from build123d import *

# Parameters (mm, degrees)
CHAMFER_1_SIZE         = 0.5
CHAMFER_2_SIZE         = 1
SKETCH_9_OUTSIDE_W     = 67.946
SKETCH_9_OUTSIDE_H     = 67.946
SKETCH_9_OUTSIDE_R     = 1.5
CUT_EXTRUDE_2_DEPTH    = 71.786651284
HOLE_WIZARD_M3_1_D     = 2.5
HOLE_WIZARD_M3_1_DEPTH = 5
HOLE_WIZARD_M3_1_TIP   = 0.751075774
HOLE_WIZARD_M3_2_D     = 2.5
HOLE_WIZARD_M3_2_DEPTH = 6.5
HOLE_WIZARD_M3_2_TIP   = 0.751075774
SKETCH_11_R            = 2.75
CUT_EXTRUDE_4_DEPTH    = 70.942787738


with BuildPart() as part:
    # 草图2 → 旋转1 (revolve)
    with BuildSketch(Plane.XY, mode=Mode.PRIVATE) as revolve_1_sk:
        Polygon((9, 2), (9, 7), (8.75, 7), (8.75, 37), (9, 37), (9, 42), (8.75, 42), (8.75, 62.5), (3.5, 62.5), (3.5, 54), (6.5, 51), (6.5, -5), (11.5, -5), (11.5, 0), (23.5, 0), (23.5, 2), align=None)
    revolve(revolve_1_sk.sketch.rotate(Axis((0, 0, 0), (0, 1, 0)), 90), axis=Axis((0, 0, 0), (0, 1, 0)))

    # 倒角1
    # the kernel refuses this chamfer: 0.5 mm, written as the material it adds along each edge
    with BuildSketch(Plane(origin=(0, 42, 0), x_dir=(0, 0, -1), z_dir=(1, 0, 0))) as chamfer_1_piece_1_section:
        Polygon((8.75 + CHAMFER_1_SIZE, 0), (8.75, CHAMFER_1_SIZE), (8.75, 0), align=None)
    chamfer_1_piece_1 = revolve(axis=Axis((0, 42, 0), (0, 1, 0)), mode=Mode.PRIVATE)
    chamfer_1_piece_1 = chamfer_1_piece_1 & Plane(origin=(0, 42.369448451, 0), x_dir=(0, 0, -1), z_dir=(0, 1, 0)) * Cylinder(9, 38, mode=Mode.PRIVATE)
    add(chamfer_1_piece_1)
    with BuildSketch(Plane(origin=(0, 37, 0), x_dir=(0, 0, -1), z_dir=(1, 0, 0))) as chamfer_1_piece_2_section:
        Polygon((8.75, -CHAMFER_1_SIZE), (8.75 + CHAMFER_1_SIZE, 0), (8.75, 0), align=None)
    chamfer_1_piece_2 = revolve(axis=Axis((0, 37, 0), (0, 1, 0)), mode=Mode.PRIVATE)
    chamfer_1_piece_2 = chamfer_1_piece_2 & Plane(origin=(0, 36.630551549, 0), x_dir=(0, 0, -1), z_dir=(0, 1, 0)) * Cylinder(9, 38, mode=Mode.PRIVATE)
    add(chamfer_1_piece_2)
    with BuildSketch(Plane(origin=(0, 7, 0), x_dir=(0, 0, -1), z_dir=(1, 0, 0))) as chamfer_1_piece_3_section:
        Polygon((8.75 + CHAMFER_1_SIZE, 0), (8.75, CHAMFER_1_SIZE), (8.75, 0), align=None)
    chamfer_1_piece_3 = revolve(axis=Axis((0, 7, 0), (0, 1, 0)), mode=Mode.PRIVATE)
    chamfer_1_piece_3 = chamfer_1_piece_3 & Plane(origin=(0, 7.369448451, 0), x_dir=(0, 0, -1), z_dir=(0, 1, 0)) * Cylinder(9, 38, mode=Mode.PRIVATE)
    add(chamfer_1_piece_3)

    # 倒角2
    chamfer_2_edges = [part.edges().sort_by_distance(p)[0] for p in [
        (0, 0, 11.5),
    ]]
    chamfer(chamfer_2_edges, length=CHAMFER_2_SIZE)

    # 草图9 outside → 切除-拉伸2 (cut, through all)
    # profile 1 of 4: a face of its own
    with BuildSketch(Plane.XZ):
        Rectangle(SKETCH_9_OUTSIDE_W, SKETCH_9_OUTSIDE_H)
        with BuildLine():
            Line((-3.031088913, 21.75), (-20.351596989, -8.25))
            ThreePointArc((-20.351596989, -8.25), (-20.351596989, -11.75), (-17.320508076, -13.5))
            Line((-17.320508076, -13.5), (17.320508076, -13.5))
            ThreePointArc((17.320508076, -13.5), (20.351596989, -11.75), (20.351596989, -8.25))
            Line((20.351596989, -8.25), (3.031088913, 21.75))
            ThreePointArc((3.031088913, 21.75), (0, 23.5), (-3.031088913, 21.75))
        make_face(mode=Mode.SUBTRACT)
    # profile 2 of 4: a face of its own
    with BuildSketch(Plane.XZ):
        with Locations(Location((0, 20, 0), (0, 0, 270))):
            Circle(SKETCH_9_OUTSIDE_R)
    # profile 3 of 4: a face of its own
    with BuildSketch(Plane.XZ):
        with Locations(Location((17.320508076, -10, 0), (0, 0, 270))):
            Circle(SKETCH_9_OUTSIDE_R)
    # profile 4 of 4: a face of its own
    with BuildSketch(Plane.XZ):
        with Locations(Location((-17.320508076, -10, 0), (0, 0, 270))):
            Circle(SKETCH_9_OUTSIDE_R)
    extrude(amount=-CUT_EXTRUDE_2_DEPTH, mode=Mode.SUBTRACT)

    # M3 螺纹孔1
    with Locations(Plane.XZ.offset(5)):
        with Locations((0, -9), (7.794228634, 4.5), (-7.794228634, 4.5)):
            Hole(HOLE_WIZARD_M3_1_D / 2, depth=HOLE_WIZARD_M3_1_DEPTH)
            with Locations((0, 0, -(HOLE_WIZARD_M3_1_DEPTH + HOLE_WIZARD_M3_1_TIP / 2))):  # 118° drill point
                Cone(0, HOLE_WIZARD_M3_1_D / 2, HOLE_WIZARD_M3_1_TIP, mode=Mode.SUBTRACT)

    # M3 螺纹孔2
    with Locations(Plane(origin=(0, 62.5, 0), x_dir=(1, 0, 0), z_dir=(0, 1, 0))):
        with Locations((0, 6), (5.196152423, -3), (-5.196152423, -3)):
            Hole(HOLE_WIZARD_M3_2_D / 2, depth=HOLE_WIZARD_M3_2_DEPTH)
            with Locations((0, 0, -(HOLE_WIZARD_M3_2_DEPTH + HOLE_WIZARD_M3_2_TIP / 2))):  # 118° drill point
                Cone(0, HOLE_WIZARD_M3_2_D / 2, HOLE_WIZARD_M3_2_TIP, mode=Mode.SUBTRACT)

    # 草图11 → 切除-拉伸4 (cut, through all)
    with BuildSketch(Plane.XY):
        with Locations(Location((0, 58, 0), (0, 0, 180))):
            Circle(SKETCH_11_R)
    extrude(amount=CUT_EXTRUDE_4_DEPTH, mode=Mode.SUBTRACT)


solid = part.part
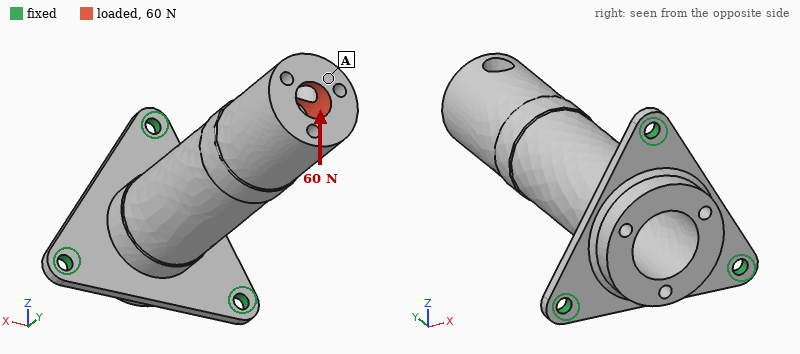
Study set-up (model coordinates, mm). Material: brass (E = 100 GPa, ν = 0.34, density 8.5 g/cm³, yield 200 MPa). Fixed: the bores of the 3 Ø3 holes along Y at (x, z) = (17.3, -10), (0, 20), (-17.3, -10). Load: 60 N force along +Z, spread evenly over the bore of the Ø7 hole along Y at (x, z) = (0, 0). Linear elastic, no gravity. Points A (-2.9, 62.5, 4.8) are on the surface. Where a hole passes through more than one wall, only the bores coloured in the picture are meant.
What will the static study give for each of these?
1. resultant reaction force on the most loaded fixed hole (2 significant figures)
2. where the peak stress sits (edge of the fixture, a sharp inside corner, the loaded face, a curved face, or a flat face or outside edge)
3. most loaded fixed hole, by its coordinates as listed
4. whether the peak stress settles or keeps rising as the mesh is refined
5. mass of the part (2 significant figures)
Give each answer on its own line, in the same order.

130 N
edge of the fixture
(0, 20)
keeps rising
88 g
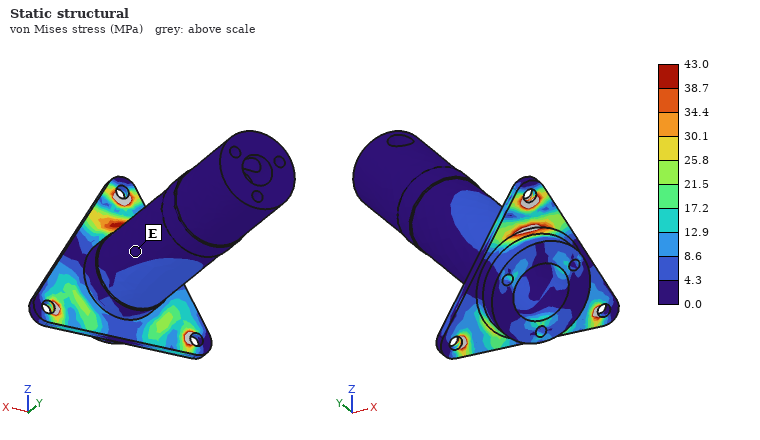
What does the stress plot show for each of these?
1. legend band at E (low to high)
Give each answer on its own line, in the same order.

0.0 to 4.3 MPa
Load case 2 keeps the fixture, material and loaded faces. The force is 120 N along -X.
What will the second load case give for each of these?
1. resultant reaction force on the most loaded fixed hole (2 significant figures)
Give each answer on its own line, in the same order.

230 N
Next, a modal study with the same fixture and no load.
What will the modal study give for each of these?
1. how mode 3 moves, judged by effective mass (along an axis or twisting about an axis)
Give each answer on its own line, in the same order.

along Y
